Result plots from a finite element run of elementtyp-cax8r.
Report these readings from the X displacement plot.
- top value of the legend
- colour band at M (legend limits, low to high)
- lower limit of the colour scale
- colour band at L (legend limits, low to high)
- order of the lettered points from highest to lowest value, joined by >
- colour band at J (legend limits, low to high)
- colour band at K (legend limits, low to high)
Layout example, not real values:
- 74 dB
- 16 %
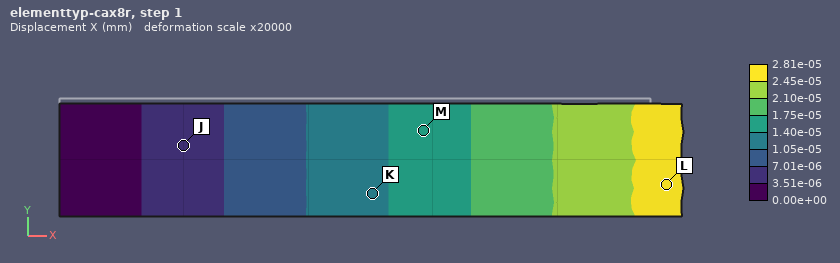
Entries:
- 2.81e-05 mm
- 1.40e-05 to 1.75e-05 mm
- 0.00e+00 mm
- 2.45e-05 to 2.81e-05 mm
- L > M > K > J
- 3.51e-06 to 7.01e-06 mm
- 1.05e-05 to 1.40e-05 mm
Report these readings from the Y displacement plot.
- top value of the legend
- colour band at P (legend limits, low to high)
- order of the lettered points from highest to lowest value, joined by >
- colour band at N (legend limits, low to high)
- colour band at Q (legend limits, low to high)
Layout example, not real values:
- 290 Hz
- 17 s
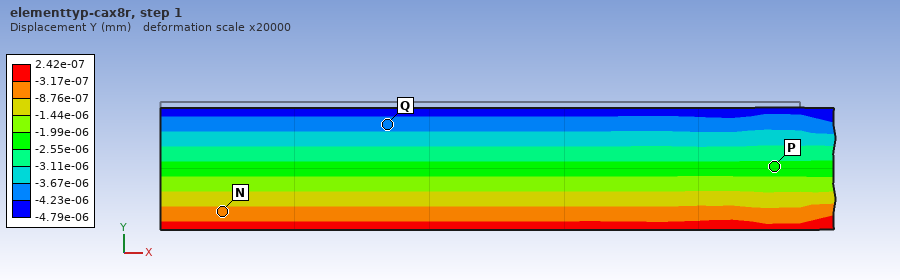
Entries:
- 2.42e-07 mm
- -2.55e-06 to -1.99e-06 mm
- N > P > Q
- -8.76e-07 to -3.17e-07 mm
- -4.23e-06 to -3.67e-06 mm
